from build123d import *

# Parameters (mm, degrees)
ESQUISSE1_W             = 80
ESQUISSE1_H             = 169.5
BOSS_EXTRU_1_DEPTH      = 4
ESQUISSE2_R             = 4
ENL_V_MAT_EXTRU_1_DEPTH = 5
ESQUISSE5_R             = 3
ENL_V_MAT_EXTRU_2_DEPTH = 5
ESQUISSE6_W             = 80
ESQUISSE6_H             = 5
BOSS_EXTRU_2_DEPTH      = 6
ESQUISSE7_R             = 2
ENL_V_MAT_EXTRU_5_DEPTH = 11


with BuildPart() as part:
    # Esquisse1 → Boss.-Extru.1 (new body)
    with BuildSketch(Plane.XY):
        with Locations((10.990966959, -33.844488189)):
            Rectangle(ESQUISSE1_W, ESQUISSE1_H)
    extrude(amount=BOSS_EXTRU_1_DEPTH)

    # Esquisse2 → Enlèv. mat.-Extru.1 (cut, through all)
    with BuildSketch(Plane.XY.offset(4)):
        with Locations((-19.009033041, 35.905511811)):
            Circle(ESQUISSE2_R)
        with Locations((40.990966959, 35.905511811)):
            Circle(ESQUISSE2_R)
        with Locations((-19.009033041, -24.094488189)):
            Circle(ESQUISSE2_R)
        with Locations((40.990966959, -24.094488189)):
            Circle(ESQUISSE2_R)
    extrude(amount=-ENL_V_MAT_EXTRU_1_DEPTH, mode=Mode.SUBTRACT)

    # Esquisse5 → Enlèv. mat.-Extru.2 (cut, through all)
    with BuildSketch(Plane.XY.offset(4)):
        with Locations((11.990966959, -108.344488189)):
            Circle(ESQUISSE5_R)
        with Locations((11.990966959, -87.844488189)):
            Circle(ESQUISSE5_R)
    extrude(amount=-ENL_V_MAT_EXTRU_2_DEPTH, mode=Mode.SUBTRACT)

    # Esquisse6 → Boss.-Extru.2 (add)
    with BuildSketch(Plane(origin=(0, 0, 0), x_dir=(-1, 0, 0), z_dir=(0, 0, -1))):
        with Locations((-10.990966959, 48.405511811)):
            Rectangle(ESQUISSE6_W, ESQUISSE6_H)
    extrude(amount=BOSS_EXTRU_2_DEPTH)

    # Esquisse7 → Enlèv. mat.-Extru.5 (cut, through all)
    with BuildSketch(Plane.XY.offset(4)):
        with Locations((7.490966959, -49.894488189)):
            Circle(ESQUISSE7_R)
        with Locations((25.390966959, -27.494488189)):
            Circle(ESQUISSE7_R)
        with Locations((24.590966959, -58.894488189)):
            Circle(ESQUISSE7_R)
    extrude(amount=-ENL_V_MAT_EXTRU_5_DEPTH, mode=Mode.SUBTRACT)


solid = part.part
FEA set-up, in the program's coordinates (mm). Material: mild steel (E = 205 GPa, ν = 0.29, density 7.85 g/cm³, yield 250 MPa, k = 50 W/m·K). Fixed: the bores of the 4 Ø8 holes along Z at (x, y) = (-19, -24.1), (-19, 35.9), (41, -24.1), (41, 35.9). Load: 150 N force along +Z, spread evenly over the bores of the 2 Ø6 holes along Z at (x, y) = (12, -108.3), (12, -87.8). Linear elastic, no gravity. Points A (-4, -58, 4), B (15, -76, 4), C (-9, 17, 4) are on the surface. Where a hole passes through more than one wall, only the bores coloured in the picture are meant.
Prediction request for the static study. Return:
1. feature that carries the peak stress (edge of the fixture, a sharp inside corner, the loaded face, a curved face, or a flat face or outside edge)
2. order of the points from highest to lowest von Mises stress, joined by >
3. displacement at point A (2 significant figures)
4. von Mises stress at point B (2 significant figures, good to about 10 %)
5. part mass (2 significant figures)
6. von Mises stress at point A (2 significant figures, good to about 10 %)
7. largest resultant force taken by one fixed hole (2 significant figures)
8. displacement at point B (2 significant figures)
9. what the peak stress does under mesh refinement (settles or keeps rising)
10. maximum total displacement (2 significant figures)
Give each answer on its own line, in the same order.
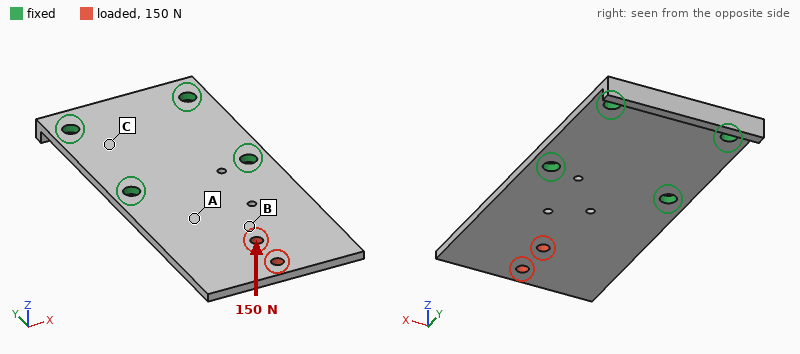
edge of the fixture
A > B > C
0.066 mm
19 MPa
440 g
28 MPa
93 N
0.14 mm
keeps rising
0.34 mm
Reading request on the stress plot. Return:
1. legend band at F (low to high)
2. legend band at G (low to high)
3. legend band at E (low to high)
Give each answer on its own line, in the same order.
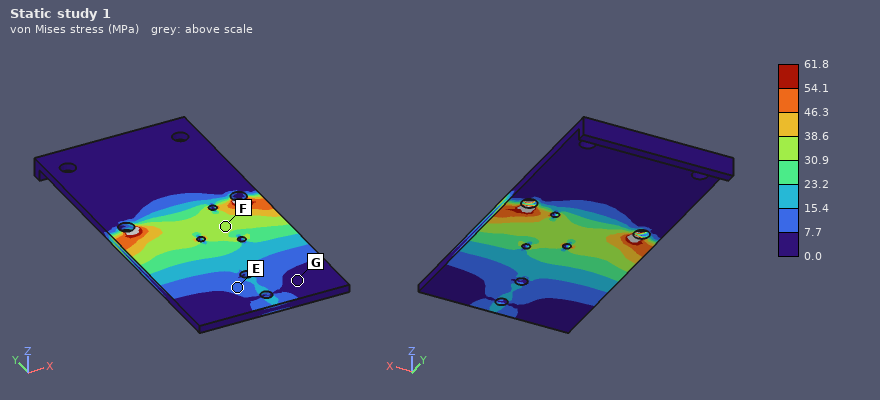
30.9 to 38.6 MPa
0.0 to 7.7 MPa
7.7 to 15.4 MPa
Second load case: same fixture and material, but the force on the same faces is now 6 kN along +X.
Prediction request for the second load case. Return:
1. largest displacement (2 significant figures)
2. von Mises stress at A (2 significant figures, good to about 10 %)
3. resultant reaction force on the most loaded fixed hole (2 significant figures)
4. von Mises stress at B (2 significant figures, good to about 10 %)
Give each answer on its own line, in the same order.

59 µm
47 MPa
7.3 kN
50 MPa
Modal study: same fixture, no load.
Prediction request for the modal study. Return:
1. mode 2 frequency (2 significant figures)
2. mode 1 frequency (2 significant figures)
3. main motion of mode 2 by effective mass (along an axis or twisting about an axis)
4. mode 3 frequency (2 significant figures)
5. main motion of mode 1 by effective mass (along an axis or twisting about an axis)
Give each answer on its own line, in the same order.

1100 Hz
370 Hz
twisting about Y
2300 Hz
along Z
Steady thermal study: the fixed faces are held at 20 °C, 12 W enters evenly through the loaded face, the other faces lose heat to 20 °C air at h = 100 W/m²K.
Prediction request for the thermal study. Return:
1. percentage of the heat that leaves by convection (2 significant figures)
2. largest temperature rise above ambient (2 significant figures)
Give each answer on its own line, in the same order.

91 %
22 K
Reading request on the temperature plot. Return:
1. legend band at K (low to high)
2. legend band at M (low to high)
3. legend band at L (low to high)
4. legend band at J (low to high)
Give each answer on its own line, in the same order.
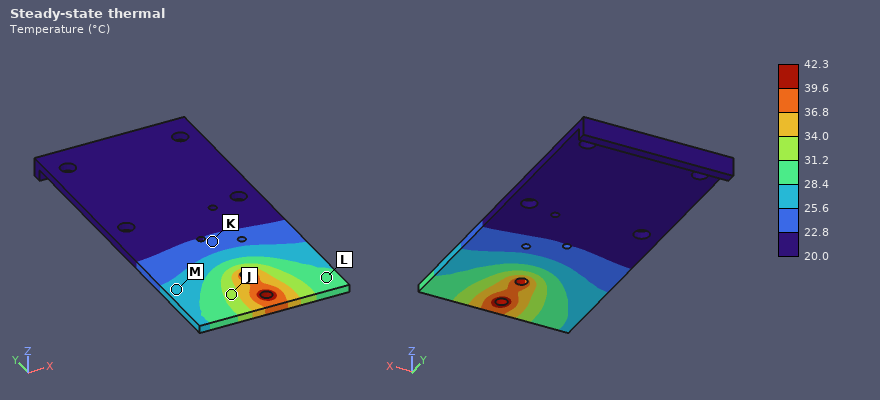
22.8 to 25.6 °C
25.6 to 28.4 °C
28.4 to 31.2 °C
31.2 to 34.0 °C
